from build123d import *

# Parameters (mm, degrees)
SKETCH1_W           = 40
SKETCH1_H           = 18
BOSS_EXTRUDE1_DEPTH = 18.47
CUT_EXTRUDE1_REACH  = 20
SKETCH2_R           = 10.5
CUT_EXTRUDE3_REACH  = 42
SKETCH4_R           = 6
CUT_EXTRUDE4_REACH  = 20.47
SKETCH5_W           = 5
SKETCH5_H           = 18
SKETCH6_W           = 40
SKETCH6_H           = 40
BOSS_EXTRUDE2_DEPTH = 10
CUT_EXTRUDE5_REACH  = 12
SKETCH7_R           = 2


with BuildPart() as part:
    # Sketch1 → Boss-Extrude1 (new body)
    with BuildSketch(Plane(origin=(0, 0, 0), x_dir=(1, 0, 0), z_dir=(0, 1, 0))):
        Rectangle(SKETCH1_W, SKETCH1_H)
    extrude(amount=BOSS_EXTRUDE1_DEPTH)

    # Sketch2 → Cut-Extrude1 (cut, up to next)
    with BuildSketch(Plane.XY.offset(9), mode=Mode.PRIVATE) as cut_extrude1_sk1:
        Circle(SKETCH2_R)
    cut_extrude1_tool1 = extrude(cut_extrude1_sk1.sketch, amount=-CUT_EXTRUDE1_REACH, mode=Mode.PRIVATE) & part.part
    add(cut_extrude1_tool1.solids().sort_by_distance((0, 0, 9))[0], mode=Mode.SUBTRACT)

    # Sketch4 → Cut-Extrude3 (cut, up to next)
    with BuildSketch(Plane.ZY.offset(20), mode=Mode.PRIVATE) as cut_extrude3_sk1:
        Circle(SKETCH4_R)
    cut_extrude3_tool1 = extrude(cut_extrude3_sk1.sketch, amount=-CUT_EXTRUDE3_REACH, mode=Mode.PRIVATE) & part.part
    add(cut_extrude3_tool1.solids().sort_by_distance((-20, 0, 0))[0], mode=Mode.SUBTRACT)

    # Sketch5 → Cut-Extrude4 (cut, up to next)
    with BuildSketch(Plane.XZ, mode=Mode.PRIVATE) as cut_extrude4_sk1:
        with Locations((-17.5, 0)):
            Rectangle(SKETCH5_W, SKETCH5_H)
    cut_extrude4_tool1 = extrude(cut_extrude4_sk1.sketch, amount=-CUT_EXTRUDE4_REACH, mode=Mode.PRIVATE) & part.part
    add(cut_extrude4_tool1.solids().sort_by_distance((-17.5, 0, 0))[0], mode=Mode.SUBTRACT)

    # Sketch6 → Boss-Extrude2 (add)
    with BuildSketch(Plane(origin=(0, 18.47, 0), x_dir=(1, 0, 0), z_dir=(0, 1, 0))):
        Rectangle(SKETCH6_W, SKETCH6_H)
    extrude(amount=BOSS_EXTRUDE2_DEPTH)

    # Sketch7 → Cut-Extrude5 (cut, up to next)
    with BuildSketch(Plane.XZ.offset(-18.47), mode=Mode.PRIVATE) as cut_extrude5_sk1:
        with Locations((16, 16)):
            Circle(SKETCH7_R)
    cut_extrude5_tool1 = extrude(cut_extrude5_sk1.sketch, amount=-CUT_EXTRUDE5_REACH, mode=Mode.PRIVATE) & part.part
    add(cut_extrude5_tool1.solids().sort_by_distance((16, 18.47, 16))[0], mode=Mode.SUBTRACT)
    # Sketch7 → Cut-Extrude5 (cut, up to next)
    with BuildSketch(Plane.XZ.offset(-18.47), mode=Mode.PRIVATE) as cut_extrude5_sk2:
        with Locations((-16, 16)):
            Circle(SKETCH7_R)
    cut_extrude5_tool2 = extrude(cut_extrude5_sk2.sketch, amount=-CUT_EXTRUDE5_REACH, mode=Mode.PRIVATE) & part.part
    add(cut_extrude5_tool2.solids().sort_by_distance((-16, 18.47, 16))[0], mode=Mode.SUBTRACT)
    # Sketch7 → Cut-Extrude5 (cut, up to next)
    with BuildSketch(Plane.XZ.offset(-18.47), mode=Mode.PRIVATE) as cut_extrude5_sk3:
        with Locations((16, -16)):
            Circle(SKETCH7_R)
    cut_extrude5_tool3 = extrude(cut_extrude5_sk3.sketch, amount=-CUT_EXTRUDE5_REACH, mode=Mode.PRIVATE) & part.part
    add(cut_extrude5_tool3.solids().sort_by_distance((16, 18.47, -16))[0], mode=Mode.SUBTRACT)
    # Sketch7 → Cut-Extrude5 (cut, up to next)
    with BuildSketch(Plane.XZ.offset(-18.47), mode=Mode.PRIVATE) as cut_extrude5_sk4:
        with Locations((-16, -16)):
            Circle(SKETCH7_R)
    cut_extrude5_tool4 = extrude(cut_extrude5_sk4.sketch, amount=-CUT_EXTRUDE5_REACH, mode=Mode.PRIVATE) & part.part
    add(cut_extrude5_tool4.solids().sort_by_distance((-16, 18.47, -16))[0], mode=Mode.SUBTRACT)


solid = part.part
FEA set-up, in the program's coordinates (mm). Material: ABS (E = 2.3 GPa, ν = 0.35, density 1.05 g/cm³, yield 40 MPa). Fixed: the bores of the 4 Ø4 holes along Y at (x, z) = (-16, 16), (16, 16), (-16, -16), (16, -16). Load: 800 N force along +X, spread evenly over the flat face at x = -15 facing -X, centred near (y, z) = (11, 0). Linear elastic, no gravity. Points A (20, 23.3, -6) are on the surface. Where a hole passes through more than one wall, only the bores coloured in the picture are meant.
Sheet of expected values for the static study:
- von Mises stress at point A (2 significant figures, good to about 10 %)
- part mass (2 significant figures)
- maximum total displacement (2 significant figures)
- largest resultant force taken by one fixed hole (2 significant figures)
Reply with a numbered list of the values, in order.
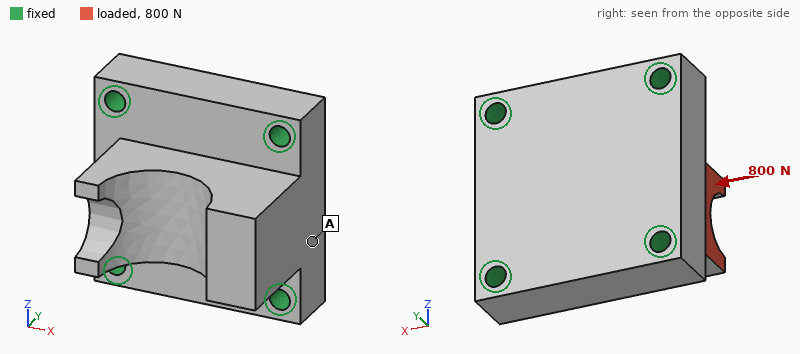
1. 2.2 MPa
2. 25 g
3. 0.20 mm
4. 280 N
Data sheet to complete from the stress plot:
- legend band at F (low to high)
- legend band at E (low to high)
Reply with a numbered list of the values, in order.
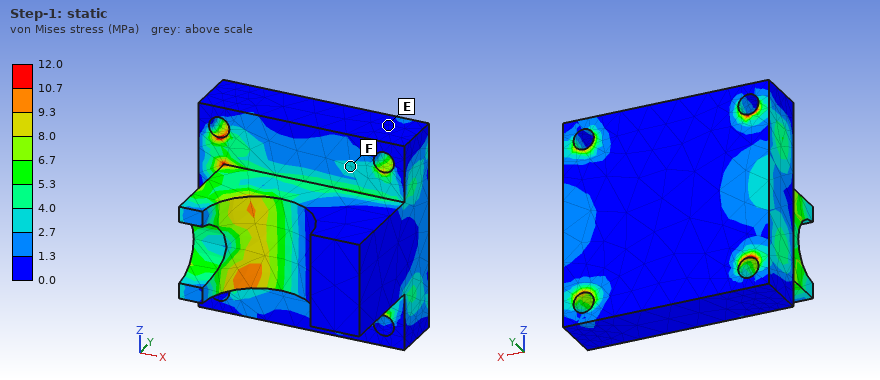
1. 2.7 to 4.0 MPa
2. 0.0 to 1.3 MPa
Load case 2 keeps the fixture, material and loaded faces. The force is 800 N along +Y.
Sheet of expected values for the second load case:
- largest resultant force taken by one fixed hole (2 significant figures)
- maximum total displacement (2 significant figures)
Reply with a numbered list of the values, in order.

1. 400 N
2. 0.21 mm
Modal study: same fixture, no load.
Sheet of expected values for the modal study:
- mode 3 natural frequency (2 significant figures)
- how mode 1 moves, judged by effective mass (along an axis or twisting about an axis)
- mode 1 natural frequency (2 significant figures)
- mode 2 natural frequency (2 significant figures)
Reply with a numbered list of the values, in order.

1. 6200 Hz
2. along X
3. 5600 Hz
4. 6200 Hz
